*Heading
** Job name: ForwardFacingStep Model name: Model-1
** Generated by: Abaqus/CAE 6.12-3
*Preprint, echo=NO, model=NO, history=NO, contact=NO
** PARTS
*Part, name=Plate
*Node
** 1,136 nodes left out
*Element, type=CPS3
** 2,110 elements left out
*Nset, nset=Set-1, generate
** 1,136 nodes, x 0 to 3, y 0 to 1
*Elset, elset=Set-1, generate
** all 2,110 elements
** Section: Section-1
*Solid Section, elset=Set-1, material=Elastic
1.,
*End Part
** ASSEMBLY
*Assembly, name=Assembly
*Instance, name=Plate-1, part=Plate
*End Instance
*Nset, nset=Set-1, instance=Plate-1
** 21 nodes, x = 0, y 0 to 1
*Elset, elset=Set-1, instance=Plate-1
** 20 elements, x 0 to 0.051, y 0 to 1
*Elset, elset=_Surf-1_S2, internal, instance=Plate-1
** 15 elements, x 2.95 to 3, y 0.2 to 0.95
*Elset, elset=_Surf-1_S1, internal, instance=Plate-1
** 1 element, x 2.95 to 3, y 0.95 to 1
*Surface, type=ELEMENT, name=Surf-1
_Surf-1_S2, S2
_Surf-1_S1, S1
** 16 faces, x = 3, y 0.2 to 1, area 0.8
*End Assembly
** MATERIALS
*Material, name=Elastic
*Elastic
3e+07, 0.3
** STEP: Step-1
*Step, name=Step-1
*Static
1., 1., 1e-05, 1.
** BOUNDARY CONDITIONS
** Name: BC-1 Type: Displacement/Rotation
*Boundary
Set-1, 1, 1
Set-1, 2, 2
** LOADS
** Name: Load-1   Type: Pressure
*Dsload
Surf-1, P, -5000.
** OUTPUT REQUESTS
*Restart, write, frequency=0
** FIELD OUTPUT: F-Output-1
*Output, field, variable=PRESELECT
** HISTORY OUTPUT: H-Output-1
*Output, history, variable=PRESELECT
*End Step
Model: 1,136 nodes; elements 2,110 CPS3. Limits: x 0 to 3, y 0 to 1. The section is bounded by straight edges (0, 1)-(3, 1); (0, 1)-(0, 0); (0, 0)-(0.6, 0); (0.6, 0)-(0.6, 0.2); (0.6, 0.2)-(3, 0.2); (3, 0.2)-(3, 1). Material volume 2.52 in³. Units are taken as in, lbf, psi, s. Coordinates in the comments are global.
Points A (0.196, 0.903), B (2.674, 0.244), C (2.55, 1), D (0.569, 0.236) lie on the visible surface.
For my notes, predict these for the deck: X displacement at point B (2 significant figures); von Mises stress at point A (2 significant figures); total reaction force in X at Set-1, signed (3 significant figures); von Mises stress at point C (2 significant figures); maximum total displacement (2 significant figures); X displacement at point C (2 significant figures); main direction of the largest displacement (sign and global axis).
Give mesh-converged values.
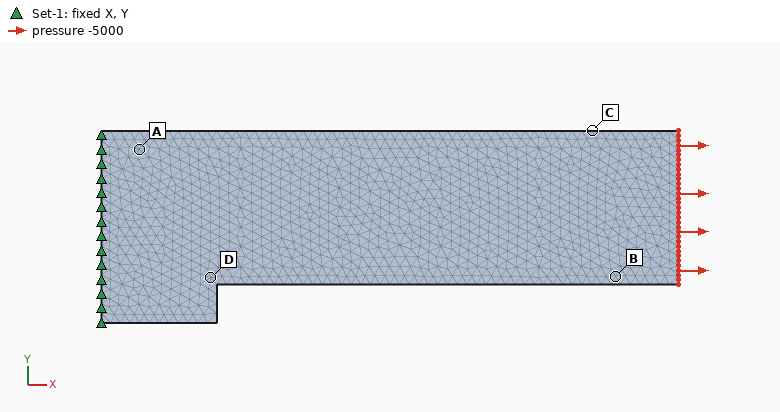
4.1e-04 in
5700 psi
-4000 lbf
5000 psi
5.6e-04 in
4.4e-04 in
+X
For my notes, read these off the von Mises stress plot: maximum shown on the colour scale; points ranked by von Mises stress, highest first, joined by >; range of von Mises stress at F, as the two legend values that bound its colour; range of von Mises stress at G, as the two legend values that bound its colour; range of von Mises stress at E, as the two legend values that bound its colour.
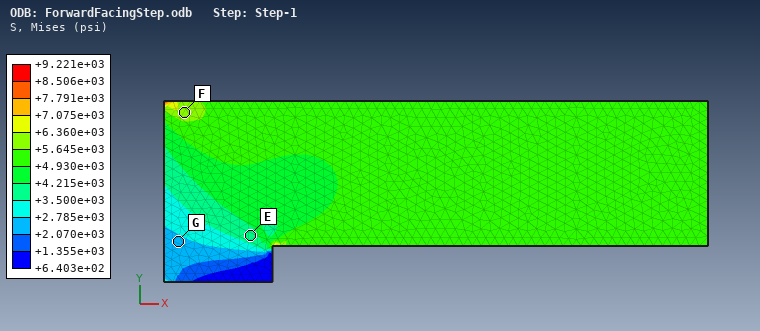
+9.221e+03 psi
F > E > G
+5.645e+03 to +6.360e+03 psi
+2.070e+03 to +2.785e+03 psi
+3.500e+03 to +4.215e+03 psi
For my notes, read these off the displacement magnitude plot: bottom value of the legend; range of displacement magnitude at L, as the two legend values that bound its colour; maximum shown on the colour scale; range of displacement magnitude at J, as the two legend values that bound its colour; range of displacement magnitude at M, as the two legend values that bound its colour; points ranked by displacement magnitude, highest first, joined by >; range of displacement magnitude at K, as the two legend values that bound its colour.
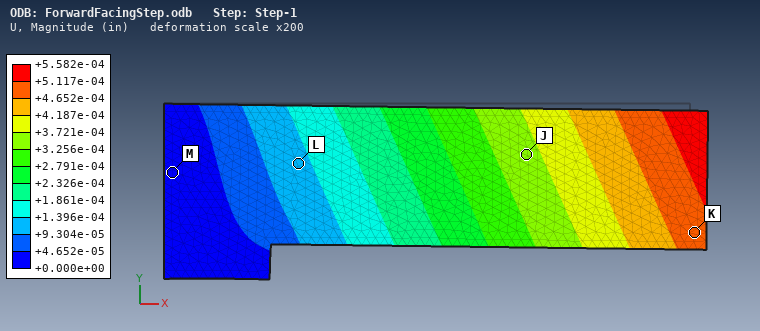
+0.000e+00 in
+9.304e-05 to +1.396e-04 in
+5.582e-04 in
+3.256e-04 to +3.721e-04 in
+0.000e+00 to +4.652e-05 in
K > J > L > M
+4.652e-04 to +5.117e-04 in
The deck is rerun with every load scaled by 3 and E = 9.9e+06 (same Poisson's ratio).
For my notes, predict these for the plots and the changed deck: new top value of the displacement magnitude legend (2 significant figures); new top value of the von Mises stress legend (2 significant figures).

0.0051 in
28000 psi
